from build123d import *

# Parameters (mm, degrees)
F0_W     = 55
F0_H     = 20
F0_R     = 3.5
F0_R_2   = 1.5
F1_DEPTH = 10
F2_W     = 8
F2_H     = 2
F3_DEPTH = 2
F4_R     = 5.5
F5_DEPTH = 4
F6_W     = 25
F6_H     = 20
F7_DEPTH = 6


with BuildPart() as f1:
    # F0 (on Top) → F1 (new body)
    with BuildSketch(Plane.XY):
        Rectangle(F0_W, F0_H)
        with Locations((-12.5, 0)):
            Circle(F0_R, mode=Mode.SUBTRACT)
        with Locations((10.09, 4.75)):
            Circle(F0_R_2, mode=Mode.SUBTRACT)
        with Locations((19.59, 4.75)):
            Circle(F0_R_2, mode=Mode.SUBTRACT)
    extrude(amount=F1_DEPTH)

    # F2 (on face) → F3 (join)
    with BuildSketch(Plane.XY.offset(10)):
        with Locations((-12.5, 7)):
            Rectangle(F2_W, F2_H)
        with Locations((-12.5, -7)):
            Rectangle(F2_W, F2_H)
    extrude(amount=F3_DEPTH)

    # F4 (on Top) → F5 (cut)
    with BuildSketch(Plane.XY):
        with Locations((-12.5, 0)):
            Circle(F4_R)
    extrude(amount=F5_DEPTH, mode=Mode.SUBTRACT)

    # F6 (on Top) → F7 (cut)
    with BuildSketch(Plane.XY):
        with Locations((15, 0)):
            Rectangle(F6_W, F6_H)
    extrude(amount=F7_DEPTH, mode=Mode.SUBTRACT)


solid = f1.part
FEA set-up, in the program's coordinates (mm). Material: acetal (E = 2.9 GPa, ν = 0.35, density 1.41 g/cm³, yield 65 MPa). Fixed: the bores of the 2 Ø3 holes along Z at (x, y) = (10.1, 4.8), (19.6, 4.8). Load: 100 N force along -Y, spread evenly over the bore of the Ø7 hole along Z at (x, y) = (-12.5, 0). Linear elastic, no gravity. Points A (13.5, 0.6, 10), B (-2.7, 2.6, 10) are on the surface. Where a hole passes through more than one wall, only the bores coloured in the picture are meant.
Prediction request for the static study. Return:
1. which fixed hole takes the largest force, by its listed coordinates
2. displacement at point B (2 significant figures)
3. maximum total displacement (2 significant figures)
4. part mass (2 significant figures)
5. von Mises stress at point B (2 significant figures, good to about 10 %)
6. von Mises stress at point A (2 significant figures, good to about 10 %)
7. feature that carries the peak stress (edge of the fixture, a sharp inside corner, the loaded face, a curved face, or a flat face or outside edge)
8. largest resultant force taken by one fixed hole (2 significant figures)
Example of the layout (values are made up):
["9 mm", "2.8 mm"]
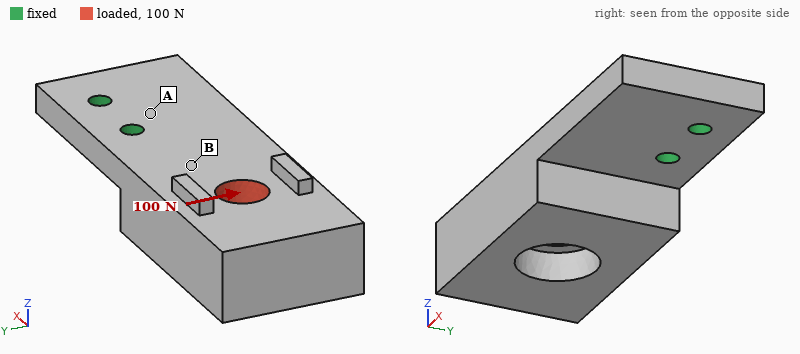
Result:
["(10.1, 4.8)", "0.087 mm", "0.29 mm", "10 g", "3.1 MPa", "6.6 MPa", "edge of the fixture", "270 N"]
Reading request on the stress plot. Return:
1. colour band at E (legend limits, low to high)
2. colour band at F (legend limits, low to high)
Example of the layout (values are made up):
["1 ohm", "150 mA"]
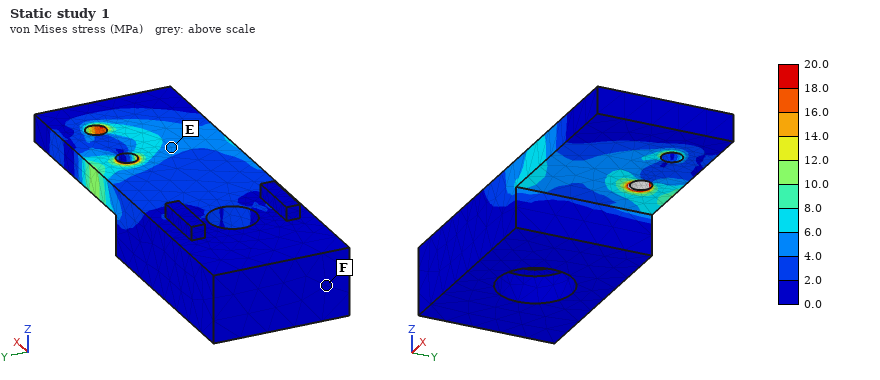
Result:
["4.0 to 6.0 MPa", "0.0 to 2.0 MPa"]
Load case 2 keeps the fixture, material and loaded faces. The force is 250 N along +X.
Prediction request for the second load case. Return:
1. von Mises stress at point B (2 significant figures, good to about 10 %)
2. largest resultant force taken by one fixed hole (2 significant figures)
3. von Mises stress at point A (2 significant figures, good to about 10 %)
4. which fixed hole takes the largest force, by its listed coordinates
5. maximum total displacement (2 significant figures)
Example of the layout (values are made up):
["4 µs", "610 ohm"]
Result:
["2.6 MPa", "200 N", "3.7 MPa", "(10.1, 4.8)", "0.28 mm"]
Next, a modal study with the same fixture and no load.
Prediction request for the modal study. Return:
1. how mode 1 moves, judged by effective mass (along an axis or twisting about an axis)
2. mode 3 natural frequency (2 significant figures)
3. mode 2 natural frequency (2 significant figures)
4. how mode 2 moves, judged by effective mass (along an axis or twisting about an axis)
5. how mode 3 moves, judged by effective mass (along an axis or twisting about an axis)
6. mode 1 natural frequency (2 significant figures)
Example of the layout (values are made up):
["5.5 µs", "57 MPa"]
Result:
["along Z", "1700 Hz", "1200 Hz", "along Y", "twisting about X", "460 Hz"]
